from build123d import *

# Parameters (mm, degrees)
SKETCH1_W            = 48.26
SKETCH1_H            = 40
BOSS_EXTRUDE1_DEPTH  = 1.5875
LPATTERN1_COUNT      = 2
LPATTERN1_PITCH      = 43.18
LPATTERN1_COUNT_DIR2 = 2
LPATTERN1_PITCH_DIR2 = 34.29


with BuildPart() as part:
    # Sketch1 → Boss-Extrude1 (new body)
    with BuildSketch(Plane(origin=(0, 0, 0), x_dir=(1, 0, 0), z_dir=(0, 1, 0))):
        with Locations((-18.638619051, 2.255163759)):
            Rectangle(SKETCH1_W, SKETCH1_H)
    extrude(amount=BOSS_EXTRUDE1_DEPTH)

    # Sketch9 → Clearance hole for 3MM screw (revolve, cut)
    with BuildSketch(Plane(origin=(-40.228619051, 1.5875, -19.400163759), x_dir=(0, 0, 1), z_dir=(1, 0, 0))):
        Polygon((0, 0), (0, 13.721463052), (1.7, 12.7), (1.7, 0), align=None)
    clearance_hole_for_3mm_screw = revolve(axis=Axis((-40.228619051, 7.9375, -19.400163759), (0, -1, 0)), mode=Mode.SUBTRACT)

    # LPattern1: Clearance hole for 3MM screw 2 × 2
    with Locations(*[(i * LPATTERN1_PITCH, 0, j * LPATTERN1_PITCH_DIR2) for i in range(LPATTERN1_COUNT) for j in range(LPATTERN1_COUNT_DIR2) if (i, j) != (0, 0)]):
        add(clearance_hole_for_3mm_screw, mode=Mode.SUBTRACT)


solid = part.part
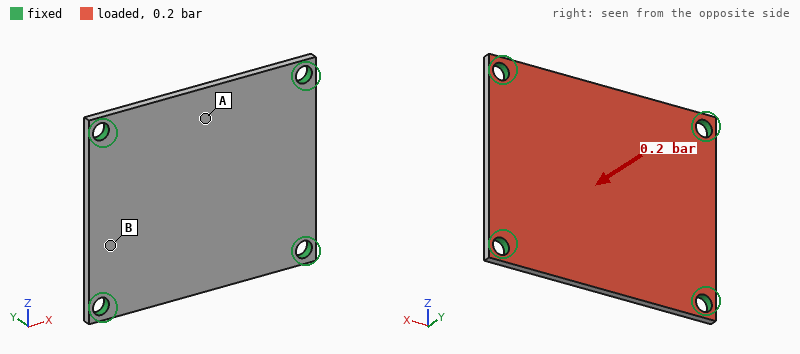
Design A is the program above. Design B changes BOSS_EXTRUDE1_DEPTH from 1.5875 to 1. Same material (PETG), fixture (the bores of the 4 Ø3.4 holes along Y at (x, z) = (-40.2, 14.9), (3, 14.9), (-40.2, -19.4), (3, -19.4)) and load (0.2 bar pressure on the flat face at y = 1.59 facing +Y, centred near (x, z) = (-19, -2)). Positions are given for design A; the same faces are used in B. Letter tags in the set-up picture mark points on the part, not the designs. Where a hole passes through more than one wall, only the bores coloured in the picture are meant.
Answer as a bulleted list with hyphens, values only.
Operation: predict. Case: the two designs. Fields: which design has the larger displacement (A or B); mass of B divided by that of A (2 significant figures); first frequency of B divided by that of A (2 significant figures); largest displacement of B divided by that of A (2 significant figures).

- B
- 0.63
- 0.64
- 3.8
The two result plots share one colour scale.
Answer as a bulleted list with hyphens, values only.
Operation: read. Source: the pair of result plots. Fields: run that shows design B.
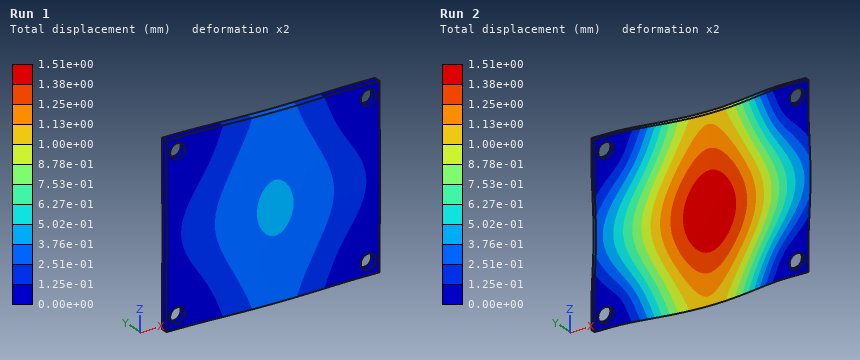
- Run 2
